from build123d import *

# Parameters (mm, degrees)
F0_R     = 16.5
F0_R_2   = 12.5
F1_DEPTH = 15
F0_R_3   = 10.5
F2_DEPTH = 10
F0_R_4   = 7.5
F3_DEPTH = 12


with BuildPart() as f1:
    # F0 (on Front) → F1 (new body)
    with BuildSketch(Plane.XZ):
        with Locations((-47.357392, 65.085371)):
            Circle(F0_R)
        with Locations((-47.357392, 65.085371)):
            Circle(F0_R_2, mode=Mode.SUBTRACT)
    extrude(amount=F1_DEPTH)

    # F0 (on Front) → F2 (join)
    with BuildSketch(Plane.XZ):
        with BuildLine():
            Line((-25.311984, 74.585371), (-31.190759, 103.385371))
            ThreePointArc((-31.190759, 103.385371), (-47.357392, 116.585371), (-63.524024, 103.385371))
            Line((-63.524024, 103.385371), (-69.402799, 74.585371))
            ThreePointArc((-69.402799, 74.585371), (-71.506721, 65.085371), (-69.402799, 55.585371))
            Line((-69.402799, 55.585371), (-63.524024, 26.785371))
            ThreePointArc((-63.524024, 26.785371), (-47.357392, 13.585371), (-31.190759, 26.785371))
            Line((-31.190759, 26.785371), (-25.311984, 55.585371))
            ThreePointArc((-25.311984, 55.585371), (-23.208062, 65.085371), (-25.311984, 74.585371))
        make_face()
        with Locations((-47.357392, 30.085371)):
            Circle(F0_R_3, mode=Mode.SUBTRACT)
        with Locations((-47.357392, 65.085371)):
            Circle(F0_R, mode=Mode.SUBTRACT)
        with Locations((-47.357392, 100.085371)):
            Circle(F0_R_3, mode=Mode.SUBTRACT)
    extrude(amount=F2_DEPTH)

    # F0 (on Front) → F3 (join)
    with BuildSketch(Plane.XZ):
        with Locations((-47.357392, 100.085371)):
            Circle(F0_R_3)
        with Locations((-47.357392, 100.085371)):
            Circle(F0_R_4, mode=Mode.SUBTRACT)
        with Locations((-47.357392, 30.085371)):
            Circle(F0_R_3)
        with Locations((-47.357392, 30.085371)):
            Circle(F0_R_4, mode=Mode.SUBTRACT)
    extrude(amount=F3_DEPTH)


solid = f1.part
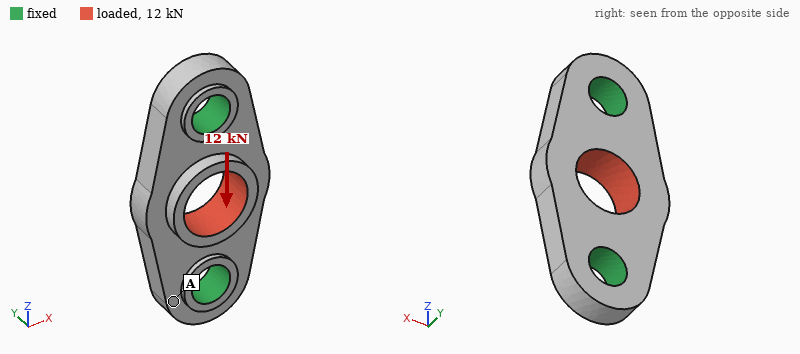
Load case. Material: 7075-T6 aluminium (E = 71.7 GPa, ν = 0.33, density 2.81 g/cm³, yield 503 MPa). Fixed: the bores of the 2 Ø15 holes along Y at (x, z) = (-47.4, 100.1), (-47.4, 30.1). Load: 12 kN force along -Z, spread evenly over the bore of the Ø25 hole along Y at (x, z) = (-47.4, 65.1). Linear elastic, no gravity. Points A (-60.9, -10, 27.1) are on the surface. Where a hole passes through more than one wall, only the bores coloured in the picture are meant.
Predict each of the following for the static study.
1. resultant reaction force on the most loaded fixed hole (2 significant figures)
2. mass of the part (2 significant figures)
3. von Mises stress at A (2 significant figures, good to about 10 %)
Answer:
6.0 kN
88 g
6.3 MPa
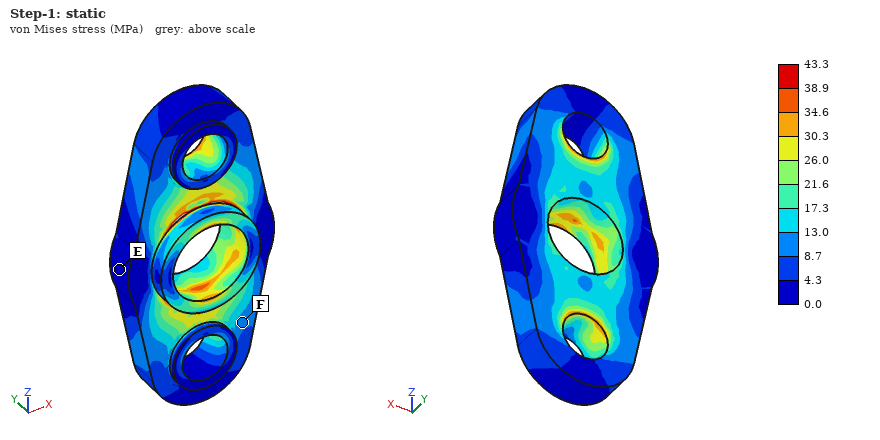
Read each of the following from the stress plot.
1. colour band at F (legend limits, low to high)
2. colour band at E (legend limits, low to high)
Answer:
8.7 to 13.0 MPa
0.0 to 4.3 MPa
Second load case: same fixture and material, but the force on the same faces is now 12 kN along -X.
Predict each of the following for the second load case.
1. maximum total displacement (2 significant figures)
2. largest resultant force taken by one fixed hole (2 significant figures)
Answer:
33 µm
6.0 kN
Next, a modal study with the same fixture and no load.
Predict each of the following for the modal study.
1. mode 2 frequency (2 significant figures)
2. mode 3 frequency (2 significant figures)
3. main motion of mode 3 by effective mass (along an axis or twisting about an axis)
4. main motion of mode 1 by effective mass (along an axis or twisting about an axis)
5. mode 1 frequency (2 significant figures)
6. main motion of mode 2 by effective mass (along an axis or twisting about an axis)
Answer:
12 kHz
21 kHz
along X
twisting about Z
11 kHz
along Y
